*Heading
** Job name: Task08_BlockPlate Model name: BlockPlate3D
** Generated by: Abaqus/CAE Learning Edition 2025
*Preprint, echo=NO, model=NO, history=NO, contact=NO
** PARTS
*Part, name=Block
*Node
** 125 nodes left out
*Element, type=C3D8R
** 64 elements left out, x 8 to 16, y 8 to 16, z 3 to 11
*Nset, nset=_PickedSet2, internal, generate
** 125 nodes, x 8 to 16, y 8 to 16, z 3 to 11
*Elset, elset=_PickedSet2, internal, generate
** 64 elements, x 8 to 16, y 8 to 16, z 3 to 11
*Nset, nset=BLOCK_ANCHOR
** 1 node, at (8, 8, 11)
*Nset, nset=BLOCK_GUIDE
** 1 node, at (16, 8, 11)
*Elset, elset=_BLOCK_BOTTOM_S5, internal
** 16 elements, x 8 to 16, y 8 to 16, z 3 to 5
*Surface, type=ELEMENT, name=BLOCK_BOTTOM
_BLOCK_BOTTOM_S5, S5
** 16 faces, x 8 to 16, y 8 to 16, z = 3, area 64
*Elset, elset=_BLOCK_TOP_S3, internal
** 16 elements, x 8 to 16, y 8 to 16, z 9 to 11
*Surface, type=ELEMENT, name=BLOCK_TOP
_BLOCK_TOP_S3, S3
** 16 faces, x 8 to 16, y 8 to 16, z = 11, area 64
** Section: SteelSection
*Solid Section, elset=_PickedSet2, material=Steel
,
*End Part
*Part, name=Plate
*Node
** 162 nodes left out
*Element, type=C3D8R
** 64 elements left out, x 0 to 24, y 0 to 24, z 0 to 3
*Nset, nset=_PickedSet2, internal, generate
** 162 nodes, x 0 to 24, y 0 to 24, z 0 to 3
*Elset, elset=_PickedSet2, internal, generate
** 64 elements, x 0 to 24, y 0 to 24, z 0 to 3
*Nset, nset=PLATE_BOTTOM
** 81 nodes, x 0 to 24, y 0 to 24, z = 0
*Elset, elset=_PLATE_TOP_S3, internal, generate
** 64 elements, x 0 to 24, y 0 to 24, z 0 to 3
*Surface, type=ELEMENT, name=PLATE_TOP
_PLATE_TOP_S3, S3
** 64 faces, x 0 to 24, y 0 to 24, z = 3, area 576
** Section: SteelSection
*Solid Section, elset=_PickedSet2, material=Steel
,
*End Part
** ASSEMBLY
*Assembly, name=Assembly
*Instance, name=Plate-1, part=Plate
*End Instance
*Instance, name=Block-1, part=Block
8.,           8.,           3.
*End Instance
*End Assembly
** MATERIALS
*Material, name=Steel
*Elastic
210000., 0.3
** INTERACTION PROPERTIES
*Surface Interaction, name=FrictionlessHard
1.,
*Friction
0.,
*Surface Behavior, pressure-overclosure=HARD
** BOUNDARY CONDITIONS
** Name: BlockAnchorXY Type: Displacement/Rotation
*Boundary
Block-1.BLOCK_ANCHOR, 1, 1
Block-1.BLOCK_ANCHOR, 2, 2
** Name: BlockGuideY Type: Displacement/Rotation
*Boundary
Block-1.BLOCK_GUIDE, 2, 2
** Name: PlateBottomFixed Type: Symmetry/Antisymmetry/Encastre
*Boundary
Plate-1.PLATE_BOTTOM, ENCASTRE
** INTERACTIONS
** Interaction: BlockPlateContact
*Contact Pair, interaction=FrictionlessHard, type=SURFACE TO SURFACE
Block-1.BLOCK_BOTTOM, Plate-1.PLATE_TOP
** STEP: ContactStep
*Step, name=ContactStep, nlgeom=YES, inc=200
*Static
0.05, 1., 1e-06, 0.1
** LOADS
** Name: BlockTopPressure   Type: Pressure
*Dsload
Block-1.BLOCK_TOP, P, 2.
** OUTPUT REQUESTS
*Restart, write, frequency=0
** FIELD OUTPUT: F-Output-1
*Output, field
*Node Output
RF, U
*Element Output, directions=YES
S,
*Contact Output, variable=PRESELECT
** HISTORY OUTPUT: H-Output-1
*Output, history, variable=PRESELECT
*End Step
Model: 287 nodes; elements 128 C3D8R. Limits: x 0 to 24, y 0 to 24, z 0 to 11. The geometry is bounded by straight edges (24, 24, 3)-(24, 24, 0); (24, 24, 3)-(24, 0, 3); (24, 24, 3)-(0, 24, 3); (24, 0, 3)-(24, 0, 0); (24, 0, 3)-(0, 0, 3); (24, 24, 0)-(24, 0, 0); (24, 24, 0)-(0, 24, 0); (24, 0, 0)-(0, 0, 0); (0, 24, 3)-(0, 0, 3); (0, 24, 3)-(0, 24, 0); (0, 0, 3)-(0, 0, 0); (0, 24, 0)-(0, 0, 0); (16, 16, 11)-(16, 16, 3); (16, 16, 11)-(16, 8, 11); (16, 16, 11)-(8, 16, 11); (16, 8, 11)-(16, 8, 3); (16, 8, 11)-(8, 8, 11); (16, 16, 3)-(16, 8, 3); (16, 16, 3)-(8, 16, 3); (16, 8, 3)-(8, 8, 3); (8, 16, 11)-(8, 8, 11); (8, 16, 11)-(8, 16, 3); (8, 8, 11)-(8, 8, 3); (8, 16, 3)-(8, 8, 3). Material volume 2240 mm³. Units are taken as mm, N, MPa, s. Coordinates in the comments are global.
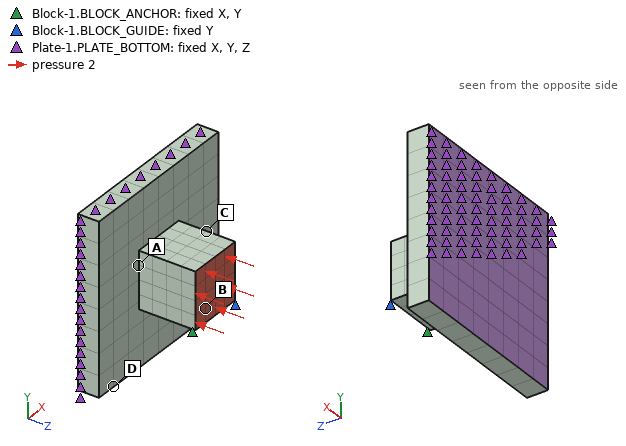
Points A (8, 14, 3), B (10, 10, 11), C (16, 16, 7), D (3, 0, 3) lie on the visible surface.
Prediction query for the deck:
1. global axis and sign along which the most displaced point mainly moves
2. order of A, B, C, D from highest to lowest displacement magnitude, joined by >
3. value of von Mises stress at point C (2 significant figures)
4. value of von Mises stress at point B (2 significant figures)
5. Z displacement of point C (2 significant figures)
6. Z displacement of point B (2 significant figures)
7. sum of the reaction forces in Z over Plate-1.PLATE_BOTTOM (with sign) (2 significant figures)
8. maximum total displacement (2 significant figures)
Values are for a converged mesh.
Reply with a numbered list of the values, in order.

1. -Z
2. B > C > A > D
3. 2.1 MPa
4. 2.0 MPa
5. -5.5e-05 mm
6. -9.3e-05 mm
7. 130 N
8. 9.9e-05 mm
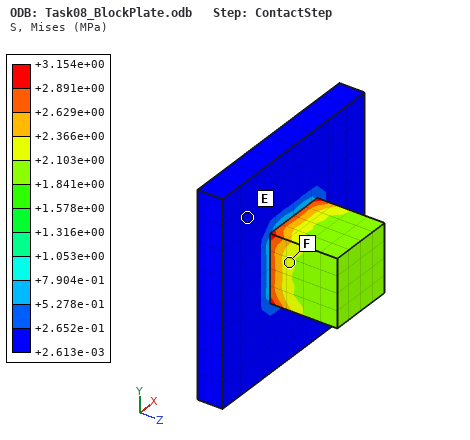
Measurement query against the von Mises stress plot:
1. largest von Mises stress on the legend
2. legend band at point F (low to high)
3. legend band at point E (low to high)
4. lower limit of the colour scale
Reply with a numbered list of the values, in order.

1. +3.154e+00 MPa
2. +2.103e+00 to +2.366e+00 MPa
3. +2.613e-03 to +2.652e-01 MPa
4. +2.613e-03 MPa
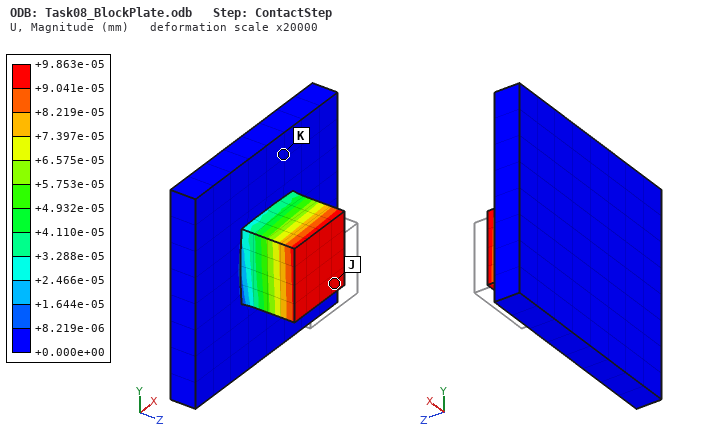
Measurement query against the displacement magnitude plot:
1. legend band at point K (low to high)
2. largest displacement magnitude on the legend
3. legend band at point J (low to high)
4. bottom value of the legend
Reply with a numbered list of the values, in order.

1. +0.000e+00 to +8.219e-06 mm
2. +9.863e-05 mm
3. +9.041e-05 to +9.863e-05 mm
4. +0.000e+00 mm
